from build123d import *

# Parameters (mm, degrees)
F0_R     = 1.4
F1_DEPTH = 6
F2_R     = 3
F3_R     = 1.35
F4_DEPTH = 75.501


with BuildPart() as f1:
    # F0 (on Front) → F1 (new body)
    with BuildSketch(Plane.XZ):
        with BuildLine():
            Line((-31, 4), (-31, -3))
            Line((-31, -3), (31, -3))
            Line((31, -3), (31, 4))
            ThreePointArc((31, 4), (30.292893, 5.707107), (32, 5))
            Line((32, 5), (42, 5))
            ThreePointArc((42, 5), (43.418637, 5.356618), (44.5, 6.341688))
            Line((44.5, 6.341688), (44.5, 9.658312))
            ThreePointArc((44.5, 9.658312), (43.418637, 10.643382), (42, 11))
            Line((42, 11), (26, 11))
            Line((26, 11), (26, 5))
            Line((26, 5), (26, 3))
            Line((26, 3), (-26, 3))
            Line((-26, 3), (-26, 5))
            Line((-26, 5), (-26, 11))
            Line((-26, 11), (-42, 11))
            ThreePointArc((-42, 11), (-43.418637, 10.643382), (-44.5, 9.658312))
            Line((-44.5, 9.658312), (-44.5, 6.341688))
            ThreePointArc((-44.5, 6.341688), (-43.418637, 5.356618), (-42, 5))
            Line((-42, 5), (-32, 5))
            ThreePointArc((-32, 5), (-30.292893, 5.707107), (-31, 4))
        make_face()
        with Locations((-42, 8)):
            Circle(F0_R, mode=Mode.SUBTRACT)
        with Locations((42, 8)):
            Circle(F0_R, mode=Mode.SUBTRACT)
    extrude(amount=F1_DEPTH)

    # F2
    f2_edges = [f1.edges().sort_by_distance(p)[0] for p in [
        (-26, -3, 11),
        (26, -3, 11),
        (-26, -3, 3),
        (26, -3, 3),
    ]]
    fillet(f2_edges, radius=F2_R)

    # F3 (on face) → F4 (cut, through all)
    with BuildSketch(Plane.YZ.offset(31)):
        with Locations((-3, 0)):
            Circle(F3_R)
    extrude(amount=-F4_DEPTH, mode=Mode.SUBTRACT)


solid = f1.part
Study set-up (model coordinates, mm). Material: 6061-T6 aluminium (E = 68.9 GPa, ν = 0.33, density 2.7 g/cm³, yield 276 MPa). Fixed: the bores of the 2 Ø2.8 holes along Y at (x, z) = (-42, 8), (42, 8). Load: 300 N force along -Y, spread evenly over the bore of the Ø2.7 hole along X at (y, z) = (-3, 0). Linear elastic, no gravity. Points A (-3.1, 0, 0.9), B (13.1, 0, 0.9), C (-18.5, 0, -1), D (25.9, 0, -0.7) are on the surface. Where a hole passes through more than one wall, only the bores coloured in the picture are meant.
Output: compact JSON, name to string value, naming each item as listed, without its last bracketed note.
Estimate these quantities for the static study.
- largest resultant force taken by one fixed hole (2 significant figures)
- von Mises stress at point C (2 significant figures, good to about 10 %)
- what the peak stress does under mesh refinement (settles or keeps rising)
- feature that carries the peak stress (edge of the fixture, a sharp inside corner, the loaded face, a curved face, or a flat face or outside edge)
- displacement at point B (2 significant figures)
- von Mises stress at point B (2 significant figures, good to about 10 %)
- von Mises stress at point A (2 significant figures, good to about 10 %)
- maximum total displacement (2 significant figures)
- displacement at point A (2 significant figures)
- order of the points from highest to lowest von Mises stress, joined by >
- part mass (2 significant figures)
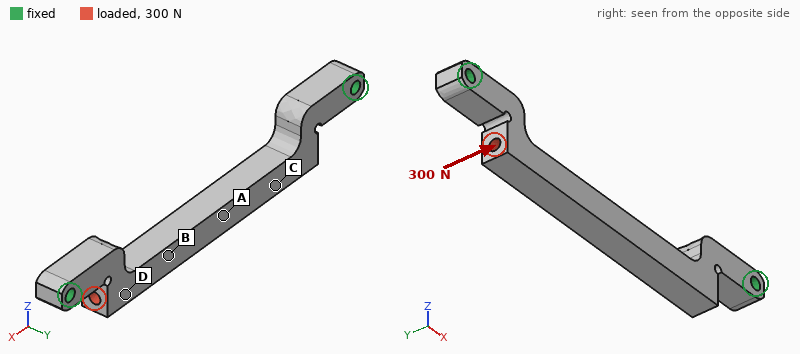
{"largest resultant force taken by one fixed hole": "150 N", "von Mises stress at point C": "17 MPa", "what the peak stress does under mesh refinement": "keeps rising", "feature that carries the peak stress": "edge of the fixture", "displacement at point B": "0.10 mm", "von Mises stress at point B": "29 MPa", "von Mises stress at point A": "40 MPa", "maximum total displacement": "0.13 mm", "displacement at point A": "0.12 mm", "order of the points from highest to lowest von Mises stress, joined by >": "A > B > C > D", "part mass": "8.6 g"}
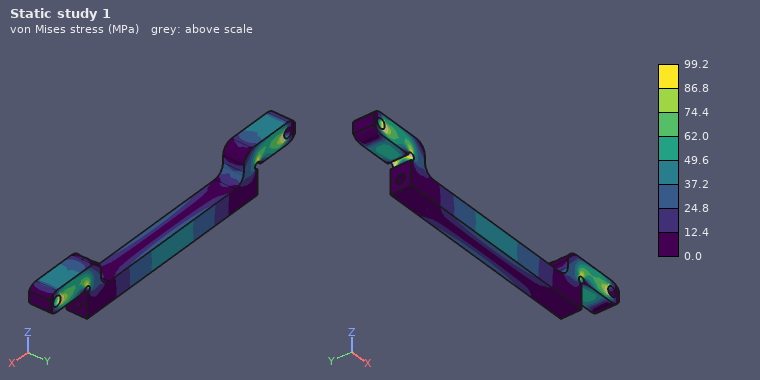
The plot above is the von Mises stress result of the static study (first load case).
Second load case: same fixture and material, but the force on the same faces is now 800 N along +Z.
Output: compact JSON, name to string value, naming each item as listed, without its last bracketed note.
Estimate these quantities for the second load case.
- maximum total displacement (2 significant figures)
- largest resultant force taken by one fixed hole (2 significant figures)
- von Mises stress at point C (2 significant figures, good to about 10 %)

{"maximum total displacement": "0.10 mm", "largest resultant force taken by one fixed hole": "740 N", "von Mises stress at point C": "32 MPa"}
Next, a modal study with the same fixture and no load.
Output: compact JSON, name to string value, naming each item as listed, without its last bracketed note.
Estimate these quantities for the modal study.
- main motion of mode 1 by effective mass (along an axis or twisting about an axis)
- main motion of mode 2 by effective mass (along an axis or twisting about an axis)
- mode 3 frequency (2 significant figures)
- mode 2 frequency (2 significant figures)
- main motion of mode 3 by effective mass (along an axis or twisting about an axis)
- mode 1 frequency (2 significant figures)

{"main motion of mode 1 by effective mass": "along Y", "main motion of mode 2 by effective mass": "along Z", "mode 3 frequency": "9000 Hz", "mode 2 frequency": "6900 Hz", "main motion of mode 3 by effective mass": "twisting about Z", "mode 1 frequency": "3800 Hz"}
